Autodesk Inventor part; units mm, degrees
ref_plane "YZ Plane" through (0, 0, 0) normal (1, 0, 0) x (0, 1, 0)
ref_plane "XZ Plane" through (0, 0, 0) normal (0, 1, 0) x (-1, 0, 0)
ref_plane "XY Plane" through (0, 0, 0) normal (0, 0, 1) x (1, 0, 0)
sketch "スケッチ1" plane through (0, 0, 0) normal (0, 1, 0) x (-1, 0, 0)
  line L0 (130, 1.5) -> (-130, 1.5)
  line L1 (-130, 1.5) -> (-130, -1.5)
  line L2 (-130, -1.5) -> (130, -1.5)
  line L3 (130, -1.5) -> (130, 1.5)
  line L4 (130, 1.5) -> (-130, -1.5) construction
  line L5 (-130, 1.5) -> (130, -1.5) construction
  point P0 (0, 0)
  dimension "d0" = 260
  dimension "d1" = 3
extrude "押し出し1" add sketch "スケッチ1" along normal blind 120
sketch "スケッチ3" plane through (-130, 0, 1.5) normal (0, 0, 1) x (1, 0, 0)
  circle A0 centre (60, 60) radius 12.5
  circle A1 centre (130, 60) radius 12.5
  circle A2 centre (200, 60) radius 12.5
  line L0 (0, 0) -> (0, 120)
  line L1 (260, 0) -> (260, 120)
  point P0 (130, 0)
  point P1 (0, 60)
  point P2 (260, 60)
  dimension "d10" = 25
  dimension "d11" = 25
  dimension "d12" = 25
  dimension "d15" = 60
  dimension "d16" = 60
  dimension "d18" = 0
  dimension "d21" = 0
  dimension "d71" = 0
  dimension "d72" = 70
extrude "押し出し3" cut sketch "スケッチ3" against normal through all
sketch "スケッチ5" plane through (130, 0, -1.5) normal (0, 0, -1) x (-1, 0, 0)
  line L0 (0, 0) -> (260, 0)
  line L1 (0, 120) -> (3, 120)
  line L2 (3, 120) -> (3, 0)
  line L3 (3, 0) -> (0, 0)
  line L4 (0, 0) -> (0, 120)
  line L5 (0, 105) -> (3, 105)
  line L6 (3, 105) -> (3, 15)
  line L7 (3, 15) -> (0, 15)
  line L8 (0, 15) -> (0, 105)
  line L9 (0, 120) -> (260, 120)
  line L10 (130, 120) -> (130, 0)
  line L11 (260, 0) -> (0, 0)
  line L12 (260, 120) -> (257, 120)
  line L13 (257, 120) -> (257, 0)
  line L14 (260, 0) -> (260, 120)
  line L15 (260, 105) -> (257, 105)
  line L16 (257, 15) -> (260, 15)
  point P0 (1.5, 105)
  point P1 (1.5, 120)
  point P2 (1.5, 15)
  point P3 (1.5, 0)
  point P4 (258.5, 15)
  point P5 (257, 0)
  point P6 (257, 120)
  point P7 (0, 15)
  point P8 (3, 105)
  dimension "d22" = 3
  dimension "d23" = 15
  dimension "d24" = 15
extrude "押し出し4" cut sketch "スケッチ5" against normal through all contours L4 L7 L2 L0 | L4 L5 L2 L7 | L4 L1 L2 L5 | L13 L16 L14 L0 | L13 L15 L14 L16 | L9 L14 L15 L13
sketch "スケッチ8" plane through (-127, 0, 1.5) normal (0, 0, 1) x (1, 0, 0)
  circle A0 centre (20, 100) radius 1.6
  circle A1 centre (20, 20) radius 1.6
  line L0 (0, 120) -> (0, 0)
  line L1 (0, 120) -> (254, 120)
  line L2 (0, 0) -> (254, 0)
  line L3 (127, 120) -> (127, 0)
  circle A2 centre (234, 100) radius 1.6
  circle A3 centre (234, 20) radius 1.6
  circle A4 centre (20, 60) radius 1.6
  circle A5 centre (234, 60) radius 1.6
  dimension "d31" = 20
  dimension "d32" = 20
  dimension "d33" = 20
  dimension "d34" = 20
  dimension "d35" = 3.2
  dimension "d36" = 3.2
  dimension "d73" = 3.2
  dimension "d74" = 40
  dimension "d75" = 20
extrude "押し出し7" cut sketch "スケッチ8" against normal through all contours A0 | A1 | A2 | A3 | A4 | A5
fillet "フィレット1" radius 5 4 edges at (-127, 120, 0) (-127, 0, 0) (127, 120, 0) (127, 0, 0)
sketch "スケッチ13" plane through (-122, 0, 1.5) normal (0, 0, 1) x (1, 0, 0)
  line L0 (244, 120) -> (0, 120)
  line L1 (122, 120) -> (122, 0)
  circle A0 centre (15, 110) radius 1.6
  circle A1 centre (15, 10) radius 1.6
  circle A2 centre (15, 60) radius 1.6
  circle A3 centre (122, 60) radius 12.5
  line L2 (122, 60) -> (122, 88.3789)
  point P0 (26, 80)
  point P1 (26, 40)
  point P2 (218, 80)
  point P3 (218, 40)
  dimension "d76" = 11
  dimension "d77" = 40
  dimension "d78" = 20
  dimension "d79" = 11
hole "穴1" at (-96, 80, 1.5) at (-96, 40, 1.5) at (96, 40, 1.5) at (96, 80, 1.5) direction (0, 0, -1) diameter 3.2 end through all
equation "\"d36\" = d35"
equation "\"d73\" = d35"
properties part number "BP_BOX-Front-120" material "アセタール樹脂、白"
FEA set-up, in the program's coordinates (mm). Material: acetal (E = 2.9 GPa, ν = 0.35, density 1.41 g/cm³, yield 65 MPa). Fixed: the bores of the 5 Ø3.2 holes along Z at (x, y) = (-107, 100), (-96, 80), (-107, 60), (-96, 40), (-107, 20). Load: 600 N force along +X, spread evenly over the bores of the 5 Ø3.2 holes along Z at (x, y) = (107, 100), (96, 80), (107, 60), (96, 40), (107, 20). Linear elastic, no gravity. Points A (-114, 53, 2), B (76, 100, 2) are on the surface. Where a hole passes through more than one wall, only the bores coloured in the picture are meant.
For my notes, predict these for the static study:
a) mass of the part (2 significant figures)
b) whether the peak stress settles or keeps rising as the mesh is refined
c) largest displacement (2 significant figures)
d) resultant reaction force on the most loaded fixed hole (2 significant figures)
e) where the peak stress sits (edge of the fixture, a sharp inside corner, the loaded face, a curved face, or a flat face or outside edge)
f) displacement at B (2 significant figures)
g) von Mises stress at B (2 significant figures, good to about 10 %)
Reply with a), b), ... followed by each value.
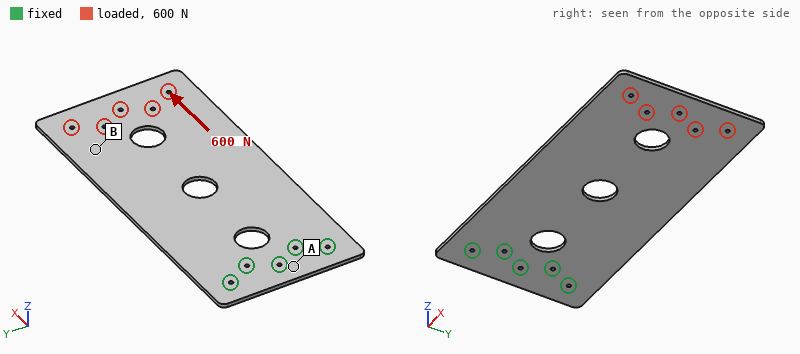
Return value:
a) 120 g
b) keeps rising
c) 0.17 mm
d) 160 N
e) edge of the fixture
f) 0.13 mm
g) 1.7 MPa
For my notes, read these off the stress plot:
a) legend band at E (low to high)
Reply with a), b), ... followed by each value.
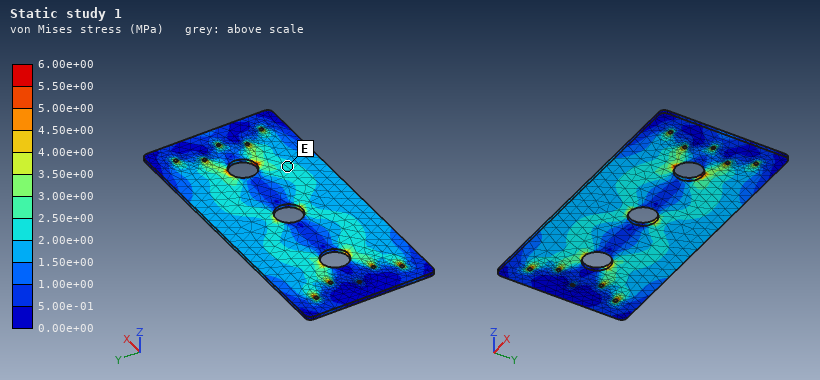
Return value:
a) 2.00e+00 to 2.50e+00 MPa
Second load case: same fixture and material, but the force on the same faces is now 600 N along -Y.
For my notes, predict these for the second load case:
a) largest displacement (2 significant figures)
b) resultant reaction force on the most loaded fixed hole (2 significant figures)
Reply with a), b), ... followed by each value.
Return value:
a) 2.8 mm
b) 1.3 kN
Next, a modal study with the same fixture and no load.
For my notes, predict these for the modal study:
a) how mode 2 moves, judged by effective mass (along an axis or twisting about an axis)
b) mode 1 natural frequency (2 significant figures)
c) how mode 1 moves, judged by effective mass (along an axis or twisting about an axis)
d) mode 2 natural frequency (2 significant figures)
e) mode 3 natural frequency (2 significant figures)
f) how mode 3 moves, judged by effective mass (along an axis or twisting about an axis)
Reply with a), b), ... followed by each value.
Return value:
a) twisting about X
b) 13 Hz
c) along Z
d) 52 Hz
e) 83 Hz
f) along Z
